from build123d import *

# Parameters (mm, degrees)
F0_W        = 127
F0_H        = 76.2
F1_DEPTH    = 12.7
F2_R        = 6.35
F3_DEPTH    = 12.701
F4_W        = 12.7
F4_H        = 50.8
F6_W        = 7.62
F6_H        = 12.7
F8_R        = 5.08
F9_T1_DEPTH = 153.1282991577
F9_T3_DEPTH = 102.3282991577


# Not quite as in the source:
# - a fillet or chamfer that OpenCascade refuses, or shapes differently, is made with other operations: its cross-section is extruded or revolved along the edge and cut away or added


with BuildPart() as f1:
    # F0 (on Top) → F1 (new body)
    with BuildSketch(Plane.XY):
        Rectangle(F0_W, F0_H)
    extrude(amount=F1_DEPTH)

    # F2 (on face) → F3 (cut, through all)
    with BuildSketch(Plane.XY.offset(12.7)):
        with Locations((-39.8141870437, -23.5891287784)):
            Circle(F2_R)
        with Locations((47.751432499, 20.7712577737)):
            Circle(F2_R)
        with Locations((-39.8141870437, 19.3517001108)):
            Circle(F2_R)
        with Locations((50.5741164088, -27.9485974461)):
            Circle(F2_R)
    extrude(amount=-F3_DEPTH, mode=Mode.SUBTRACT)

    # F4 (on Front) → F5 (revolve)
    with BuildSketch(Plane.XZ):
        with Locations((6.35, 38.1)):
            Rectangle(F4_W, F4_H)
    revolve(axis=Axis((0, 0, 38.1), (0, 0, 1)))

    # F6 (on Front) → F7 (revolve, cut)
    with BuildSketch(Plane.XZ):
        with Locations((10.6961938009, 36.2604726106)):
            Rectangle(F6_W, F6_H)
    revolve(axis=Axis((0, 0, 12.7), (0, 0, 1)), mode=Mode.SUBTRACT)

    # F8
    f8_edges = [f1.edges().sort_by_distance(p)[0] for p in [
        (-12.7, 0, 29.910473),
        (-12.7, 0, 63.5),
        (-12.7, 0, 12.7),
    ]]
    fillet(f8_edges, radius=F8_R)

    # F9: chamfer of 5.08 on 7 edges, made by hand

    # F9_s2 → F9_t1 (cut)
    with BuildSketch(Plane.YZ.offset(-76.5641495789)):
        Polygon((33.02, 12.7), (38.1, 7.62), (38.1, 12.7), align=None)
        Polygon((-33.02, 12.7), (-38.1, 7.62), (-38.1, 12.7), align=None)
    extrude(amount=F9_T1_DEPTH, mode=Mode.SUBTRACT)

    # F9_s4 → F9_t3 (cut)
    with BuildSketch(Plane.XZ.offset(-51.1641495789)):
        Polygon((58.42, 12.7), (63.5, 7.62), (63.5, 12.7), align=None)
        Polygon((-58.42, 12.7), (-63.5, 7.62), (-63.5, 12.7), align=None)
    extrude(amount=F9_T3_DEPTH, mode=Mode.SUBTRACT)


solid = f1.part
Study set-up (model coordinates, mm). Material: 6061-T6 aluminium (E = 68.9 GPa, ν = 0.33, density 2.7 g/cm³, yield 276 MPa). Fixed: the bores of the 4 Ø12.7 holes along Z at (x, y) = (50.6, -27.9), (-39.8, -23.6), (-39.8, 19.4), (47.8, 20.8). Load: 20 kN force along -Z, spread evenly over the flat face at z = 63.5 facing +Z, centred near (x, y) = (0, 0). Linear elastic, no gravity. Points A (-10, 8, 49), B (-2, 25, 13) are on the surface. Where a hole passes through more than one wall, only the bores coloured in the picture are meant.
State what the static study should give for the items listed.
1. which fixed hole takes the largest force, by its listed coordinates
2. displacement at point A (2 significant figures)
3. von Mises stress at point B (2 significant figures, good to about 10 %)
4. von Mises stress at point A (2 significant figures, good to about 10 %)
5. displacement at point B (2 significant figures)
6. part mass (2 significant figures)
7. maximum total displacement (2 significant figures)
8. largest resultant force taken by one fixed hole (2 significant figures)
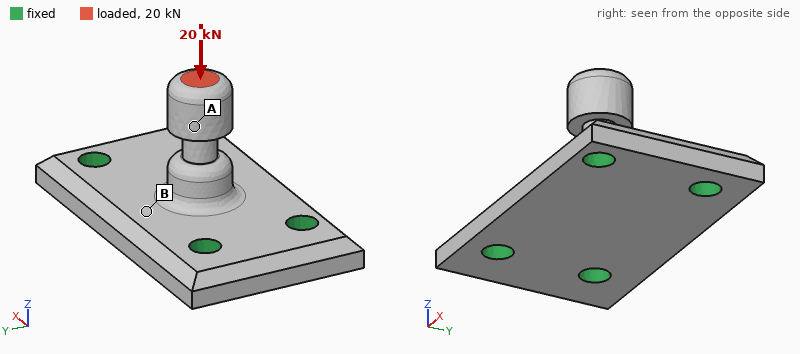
(-39.8, 19.4)
0.11 mm
45 MPa
21 MPa
0.056 mm
360 g
0.14 mm
6.2 kN
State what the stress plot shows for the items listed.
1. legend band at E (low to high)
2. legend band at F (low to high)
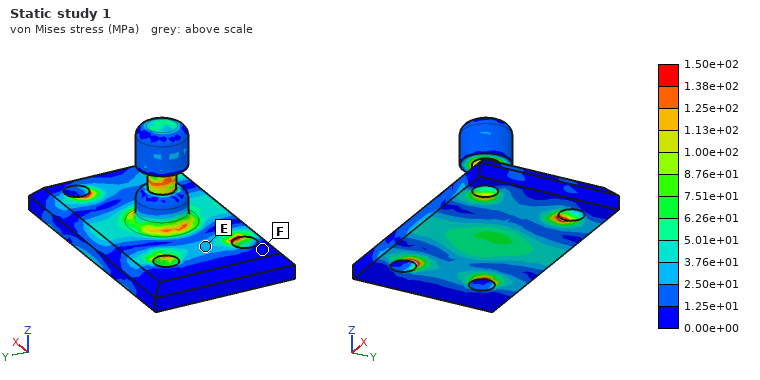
2.50e+01 to 3.76e+01 MPa
0.00e+00 to 1.25e+01 MPa
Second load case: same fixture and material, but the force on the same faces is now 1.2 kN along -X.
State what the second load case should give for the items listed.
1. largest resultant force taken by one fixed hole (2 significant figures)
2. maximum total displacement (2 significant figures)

730 N
0.19 mm
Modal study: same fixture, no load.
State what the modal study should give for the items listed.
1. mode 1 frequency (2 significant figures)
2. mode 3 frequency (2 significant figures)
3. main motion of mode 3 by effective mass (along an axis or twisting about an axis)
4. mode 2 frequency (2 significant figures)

3200 Hz
6900 Hz
along Z
3300 Hz
